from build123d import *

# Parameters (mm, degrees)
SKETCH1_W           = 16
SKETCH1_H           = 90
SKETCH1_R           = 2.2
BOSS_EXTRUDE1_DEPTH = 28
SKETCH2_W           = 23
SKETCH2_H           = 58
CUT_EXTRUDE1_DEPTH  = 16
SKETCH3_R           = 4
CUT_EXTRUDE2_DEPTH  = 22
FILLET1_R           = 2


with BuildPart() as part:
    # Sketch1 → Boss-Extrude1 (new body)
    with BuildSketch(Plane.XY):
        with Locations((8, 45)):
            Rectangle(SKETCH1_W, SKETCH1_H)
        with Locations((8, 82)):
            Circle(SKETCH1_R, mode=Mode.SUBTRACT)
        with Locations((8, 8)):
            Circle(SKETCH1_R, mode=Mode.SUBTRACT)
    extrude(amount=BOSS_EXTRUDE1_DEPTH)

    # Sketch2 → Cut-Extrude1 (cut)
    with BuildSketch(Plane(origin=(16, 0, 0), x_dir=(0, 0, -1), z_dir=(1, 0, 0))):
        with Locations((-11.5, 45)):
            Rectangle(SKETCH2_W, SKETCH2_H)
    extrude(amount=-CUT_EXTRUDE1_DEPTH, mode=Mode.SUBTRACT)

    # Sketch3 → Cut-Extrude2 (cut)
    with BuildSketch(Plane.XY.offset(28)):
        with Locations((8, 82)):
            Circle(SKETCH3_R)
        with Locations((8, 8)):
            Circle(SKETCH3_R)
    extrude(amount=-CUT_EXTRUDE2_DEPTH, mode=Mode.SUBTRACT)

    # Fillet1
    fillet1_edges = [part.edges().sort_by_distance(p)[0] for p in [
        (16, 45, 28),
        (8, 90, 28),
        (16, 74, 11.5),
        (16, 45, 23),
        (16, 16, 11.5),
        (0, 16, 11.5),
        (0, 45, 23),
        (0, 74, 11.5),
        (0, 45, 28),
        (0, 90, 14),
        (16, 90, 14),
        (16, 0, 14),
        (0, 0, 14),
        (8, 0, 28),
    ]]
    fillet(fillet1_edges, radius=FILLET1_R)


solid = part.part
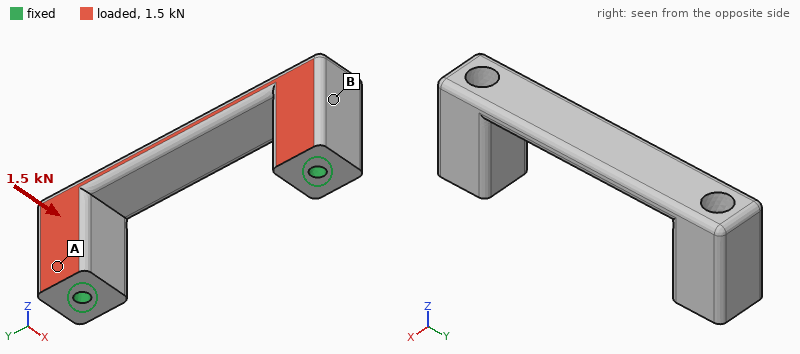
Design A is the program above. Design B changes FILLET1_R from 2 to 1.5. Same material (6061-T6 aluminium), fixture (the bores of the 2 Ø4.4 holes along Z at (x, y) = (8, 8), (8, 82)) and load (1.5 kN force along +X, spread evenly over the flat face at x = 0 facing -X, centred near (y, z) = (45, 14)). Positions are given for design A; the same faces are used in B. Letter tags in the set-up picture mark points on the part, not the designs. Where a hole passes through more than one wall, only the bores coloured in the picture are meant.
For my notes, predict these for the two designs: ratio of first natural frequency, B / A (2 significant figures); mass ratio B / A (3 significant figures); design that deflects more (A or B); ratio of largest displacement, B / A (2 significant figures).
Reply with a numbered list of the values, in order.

1. 1.00
2. 1.01
3. B
4. 1.2
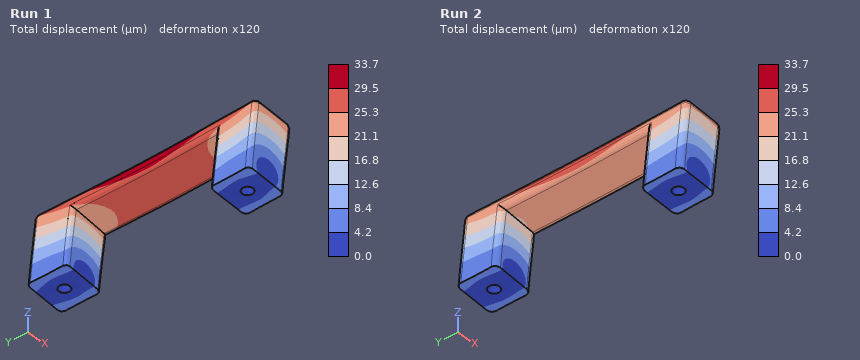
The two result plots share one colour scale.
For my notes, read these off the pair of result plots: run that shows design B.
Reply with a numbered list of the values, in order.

1. Run 1
